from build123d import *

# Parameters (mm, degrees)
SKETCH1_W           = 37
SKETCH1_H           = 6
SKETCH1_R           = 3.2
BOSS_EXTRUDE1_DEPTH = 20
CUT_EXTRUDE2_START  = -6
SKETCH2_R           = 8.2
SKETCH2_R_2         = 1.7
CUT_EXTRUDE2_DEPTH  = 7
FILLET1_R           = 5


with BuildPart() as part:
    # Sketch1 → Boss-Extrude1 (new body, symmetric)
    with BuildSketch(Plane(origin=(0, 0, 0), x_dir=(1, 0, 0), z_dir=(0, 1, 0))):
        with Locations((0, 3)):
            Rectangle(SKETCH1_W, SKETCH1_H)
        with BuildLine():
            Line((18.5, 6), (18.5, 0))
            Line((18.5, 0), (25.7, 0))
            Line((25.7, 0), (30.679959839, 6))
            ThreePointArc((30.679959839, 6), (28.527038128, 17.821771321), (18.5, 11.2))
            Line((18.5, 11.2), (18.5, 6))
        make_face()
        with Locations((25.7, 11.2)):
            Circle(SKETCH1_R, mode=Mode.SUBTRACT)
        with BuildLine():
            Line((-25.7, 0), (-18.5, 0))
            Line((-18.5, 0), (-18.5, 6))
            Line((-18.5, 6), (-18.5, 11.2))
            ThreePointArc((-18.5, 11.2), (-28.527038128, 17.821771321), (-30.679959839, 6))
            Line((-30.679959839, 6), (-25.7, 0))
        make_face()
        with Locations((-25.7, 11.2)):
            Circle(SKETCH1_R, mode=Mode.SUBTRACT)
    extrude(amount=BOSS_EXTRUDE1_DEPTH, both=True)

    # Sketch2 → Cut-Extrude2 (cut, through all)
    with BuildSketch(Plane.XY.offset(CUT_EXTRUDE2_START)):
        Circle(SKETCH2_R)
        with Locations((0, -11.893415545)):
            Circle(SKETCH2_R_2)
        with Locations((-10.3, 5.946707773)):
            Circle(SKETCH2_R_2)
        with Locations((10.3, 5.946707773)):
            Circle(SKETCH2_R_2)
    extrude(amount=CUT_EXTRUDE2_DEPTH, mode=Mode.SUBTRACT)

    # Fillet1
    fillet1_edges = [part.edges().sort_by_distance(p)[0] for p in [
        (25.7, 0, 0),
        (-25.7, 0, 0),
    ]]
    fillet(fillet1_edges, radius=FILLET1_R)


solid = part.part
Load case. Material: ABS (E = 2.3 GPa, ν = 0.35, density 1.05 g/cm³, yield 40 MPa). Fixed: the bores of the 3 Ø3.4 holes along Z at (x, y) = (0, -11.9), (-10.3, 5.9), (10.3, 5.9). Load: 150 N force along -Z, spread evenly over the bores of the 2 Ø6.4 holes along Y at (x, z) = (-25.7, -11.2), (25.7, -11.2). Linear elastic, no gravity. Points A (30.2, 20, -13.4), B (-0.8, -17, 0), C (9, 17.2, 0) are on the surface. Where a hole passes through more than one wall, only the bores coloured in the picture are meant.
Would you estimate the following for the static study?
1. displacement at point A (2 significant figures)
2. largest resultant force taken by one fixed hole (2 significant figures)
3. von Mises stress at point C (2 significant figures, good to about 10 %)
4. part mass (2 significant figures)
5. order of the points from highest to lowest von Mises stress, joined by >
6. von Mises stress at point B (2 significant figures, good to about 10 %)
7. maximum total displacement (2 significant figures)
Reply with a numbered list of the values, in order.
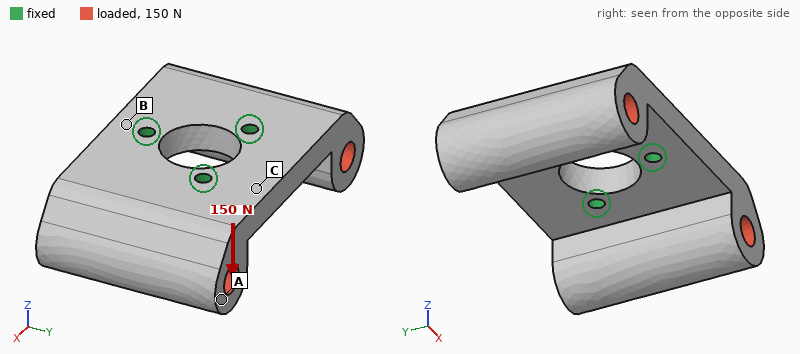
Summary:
1. 0.14 mm
2. 68 N
3. 2.5 MPa
4. 23 g
5. B > C > A
6. 3.9 MPa
7. 0.23 mm
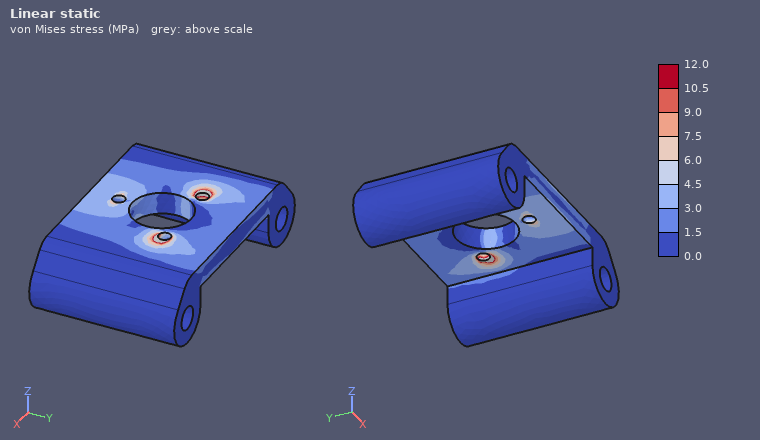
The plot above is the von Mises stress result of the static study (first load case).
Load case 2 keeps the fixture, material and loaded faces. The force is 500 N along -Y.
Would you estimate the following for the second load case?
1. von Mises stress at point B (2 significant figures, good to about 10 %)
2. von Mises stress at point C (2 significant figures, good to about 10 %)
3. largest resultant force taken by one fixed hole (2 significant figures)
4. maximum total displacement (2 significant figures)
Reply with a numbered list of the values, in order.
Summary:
1. 9.7 MPa
2. 3.0 MPa
3. 220 N
4. 0.24 mm
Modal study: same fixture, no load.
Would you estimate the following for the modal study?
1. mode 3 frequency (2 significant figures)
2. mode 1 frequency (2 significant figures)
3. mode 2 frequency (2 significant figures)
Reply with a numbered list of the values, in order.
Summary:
1. 2200 Hz
2. 1300 Hz
3. 1300 Hz
